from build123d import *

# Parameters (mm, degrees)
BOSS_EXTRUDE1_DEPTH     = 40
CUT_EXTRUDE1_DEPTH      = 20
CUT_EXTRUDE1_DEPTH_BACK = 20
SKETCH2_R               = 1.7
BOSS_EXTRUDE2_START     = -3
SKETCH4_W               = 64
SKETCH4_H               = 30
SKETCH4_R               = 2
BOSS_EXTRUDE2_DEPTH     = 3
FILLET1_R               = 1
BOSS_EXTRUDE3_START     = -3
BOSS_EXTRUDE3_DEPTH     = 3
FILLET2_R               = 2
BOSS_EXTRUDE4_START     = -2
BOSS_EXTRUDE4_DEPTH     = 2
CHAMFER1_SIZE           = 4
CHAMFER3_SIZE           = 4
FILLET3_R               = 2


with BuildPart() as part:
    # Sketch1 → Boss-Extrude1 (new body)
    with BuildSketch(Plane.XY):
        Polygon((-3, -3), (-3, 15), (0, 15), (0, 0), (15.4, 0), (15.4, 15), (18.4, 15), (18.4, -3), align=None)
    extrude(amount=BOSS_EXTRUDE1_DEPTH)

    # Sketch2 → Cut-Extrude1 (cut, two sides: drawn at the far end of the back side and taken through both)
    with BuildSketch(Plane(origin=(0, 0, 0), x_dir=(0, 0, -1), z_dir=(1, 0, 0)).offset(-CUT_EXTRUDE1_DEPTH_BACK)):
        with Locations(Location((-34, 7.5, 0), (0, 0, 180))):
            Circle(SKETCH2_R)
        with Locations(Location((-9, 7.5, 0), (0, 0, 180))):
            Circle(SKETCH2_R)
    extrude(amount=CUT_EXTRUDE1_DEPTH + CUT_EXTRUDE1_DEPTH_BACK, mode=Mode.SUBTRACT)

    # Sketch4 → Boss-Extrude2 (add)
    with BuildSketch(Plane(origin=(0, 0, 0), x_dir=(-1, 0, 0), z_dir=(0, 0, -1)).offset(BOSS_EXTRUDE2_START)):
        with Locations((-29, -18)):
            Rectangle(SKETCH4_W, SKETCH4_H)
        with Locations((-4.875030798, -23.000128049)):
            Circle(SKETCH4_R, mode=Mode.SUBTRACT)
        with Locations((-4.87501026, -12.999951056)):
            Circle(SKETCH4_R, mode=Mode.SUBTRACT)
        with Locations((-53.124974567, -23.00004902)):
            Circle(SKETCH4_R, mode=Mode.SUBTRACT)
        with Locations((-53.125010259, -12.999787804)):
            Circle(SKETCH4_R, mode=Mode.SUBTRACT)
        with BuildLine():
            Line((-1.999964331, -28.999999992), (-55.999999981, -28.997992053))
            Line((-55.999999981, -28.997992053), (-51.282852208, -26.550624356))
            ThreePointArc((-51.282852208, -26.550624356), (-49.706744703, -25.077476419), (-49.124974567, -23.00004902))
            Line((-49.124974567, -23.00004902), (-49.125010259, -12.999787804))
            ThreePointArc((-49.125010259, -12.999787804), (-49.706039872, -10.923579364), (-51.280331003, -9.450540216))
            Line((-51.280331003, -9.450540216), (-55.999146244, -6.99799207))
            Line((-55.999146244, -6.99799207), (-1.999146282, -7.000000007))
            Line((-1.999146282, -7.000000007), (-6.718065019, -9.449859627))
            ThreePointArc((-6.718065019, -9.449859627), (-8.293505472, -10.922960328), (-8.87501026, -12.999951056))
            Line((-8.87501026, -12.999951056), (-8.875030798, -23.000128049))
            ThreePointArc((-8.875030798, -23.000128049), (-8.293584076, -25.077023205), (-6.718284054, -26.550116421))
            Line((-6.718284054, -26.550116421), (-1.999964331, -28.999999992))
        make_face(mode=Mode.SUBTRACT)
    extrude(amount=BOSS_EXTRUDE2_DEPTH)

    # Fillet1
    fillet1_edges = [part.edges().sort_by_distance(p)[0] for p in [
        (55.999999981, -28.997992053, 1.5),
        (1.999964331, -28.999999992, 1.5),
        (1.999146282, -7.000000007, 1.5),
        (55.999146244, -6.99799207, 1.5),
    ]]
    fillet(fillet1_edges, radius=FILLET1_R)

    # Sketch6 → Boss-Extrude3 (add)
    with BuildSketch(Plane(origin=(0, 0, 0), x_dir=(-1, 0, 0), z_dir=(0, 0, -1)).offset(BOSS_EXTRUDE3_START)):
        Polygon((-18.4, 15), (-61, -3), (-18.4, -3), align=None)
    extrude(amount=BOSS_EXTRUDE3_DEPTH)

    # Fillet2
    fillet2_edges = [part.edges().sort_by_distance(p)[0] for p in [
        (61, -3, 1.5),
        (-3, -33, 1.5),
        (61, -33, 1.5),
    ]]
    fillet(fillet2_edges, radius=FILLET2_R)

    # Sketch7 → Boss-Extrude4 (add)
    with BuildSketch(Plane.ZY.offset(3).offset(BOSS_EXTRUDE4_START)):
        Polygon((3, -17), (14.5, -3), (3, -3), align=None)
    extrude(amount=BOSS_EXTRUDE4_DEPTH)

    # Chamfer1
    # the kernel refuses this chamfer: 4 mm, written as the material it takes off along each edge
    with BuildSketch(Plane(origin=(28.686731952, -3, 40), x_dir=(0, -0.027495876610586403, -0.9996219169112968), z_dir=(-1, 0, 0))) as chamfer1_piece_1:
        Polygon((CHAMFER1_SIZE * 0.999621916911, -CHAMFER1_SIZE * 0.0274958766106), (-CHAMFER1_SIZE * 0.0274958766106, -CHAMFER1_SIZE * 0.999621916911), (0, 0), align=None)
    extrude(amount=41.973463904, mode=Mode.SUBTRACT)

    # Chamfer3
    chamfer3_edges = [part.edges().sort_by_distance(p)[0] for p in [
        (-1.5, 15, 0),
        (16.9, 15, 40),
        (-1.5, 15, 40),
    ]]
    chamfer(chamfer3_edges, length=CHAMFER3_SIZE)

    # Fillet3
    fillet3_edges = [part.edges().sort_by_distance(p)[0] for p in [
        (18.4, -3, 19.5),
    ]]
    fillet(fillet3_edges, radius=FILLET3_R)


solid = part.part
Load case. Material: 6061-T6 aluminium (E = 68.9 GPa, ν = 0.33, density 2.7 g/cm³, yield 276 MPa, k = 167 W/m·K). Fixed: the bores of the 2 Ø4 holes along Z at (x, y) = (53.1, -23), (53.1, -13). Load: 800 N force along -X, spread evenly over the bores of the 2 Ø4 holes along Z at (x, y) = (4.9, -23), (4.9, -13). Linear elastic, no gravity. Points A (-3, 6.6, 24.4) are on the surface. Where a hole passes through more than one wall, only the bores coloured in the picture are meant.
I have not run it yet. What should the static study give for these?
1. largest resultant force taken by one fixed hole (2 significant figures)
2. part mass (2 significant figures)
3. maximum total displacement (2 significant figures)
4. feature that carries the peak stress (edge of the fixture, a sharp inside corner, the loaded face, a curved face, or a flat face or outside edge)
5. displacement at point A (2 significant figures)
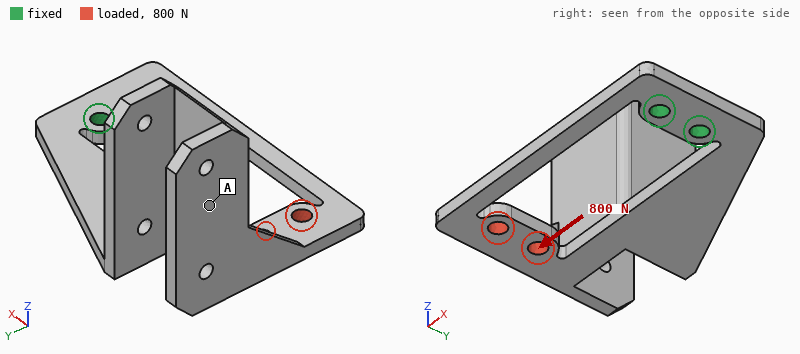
500 N
27 g
54 µm
a curved face
21 µm
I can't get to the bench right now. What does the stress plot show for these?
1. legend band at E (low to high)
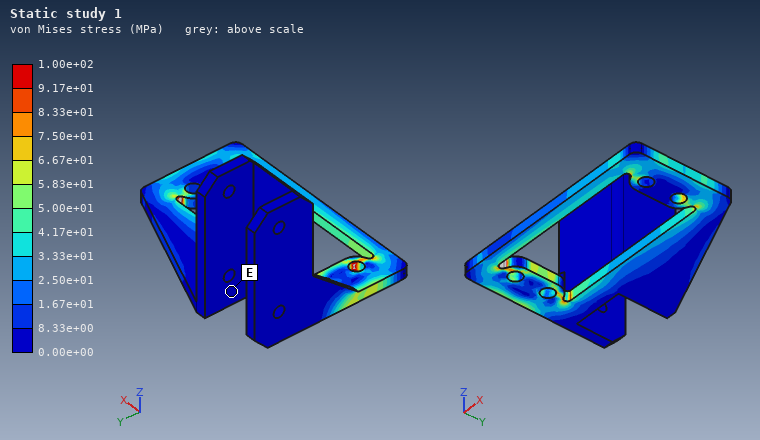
0.00e+00 to 8.33e+00 MPa
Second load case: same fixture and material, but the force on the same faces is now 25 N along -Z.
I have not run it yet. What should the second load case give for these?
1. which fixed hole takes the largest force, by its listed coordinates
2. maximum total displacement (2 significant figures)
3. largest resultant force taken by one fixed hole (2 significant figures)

(53.1, -23)
0.95 mm
16 N
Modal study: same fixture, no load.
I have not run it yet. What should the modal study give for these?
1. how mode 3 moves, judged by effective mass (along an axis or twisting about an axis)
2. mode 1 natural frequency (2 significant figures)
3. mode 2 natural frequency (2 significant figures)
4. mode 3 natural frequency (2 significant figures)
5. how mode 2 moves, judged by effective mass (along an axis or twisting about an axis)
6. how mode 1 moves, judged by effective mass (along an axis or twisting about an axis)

along Y
200 Hz
420 Hz
1100 Hz
along Y
along Z
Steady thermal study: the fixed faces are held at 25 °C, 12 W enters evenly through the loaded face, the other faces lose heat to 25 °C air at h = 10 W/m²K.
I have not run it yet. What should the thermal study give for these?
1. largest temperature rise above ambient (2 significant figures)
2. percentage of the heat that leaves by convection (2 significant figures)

81 K
31 %
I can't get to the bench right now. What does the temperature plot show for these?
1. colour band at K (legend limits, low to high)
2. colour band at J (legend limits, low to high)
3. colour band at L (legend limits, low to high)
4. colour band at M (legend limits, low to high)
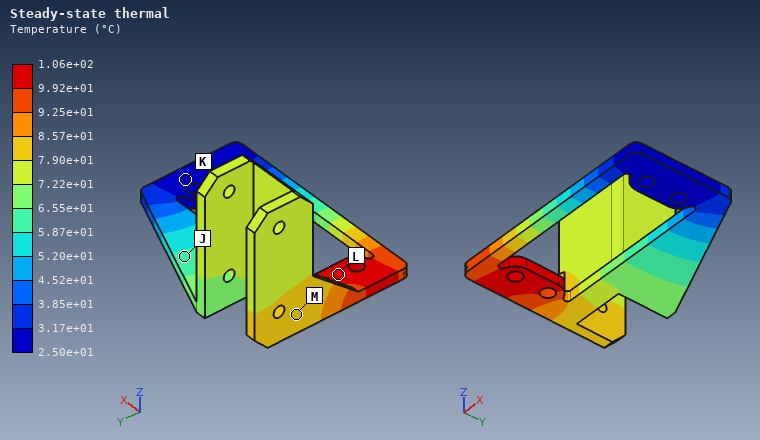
2.50e+01 to 3.17e+01 °C
5.87e+01 to 6.55e+01 °C
9.92e+01 to 1.06e+02 °C
7.90e+01 to 8.57e+01 °C
